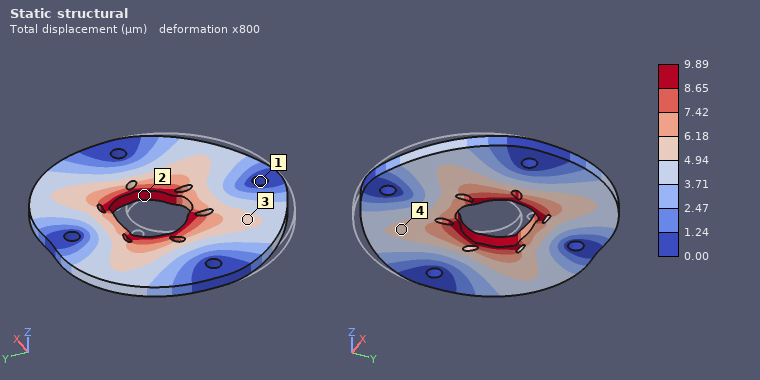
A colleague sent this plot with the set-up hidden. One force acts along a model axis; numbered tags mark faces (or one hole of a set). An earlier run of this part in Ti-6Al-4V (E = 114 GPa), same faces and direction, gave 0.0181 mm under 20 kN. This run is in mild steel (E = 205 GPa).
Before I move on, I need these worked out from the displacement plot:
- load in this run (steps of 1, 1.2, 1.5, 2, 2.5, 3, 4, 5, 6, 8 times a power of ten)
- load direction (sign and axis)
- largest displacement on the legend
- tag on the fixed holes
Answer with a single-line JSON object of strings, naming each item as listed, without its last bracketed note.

{"load in this run": "20 kN", "load direction": "+Y", "largest displacement on the legend": "9.89 µm", "tag on the fixed holes": "1"}
